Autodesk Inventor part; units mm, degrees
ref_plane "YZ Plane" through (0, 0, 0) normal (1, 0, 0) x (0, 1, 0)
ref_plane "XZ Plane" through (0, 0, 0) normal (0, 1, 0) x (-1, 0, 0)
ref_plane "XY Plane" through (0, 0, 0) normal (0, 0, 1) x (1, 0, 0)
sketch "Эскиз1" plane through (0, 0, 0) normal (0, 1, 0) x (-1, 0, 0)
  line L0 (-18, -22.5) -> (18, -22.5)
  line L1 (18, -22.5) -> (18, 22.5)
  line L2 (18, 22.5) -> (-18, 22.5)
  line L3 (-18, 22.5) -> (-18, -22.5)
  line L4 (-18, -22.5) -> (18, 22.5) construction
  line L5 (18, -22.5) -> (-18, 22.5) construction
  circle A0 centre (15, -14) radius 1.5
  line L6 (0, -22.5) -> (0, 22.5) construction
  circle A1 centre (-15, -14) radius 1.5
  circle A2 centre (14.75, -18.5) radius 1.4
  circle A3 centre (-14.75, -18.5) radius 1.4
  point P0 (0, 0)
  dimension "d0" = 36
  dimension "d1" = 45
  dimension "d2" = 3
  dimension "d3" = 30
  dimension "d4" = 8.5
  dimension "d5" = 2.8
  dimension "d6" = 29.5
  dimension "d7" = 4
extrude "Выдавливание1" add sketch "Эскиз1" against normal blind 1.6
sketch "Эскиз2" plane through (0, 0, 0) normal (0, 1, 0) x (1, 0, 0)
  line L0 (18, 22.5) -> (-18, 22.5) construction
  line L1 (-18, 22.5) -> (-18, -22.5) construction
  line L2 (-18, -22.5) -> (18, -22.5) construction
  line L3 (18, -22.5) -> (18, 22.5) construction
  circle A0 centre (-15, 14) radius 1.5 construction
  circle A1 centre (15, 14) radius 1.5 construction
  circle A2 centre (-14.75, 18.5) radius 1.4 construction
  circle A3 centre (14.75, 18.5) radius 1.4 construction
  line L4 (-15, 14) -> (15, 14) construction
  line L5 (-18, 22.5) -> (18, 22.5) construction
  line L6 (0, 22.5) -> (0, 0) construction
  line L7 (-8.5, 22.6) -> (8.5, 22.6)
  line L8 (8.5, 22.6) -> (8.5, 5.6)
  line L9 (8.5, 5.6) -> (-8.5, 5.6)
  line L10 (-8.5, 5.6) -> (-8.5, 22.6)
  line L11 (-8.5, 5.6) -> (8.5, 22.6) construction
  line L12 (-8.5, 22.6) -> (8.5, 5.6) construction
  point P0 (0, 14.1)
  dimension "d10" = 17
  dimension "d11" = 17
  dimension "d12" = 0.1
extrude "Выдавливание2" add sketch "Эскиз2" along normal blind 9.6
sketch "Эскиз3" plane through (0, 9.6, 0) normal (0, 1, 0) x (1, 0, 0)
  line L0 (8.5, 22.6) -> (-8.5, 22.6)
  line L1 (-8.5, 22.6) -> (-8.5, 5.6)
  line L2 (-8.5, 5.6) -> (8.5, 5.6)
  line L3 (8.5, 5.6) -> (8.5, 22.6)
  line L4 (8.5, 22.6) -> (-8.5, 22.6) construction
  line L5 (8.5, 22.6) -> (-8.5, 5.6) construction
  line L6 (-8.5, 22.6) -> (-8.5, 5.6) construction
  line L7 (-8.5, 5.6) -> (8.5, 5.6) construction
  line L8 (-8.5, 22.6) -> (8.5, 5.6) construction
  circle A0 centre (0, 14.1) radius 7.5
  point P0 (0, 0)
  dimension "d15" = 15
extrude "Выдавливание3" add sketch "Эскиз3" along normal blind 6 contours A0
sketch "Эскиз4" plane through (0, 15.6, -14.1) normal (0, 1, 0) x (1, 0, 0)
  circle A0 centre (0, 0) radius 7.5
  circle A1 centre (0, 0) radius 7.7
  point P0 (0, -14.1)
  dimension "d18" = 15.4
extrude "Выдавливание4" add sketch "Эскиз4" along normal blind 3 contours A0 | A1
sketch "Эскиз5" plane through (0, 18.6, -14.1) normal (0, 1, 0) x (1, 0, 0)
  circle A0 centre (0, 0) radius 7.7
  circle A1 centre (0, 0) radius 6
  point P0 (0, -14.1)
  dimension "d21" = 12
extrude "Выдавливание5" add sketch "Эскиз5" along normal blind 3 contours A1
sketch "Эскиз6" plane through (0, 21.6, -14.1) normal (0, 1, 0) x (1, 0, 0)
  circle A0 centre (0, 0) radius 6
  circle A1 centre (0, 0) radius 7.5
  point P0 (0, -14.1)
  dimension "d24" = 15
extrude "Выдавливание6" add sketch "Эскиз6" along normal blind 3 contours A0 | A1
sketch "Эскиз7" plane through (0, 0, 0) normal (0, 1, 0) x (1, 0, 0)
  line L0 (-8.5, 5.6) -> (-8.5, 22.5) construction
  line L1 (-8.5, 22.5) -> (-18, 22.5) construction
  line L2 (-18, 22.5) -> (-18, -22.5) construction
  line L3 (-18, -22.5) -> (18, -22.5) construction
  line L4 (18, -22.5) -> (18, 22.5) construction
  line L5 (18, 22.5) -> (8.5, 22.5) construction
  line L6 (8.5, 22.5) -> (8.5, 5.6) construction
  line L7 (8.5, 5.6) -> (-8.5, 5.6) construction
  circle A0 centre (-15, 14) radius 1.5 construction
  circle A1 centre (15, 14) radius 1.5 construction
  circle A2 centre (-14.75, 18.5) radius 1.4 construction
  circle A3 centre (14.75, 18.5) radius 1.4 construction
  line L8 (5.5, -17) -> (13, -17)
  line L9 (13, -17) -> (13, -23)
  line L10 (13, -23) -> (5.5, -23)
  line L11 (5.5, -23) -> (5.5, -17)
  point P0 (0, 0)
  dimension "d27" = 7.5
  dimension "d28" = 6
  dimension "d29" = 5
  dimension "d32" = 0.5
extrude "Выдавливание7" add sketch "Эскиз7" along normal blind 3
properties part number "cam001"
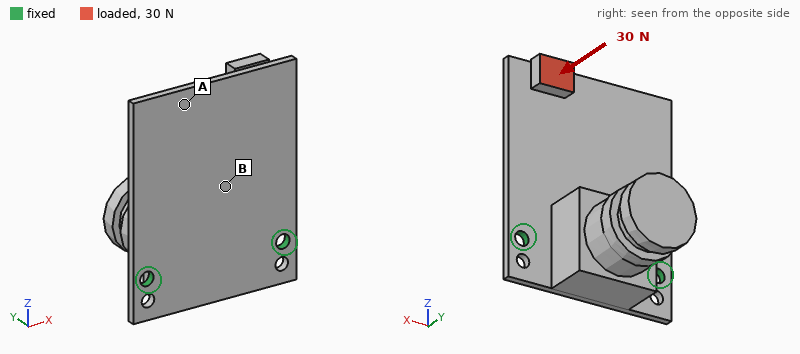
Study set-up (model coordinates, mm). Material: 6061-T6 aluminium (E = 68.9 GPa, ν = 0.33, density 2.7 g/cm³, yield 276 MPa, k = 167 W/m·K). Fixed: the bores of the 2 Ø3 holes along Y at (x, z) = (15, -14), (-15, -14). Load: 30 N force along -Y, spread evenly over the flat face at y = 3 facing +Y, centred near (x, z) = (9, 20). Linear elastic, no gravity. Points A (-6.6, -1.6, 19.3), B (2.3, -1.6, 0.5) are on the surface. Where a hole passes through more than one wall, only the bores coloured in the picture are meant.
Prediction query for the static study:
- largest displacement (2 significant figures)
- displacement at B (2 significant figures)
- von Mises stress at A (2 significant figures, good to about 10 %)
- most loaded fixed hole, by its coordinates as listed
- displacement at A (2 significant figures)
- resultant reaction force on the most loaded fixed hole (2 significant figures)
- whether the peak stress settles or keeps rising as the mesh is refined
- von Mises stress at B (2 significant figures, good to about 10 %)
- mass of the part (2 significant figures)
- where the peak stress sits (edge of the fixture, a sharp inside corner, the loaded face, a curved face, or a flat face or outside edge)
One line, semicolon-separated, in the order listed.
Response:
0.47 mm; 0.085 mm; 15 MPa; (15, -14); 0.32 mm; 29 N; keeps rising; 39 MPa; 21 g; edge of the fixture
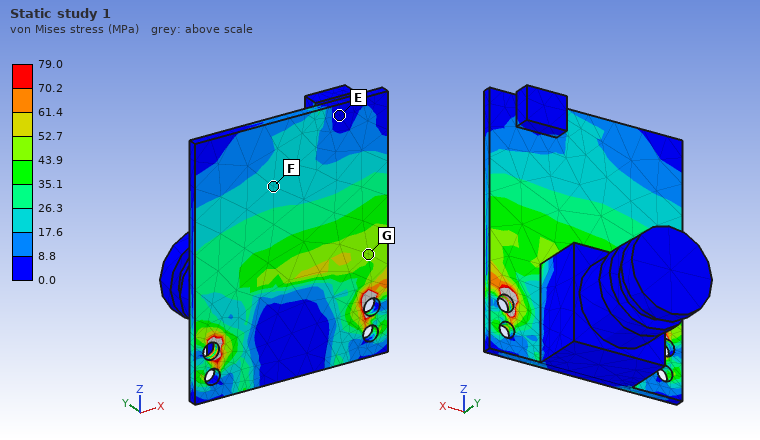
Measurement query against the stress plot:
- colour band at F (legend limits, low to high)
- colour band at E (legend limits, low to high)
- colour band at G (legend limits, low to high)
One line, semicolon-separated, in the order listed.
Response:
17.6 to 26.3 MPa; 0.0 to 8.8 MPa; 43.9 to 52.7 MPa
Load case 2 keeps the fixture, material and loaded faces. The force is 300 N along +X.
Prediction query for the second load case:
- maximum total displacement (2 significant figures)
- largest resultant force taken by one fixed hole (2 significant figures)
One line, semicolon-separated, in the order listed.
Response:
0.35 mm; 370 N
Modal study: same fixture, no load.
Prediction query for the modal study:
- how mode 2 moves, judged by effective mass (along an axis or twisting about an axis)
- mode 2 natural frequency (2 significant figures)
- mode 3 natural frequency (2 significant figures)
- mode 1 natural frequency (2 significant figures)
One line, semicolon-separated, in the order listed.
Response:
along Z; 2200 Hz; 2700 Hz; 910 Hz
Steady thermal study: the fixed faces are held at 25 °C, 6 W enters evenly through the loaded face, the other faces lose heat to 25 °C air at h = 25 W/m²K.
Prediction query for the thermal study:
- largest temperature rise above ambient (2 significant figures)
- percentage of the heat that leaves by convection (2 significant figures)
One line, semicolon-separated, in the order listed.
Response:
29 K; 17 %
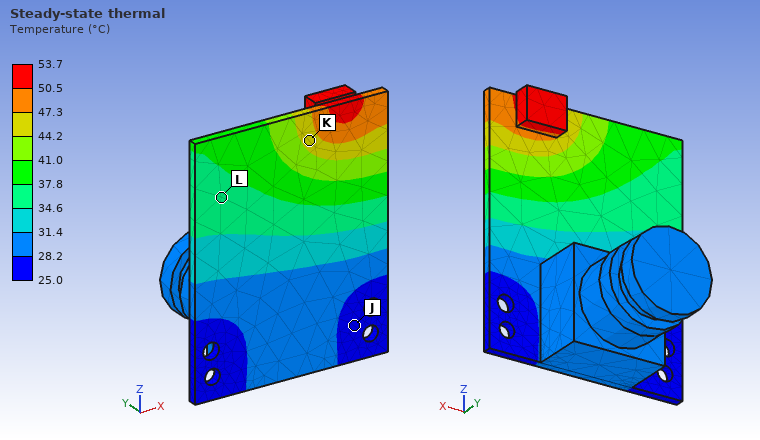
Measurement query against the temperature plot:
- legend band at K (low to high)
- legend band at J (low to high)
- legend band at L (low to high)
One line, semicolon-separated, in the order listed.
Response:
44.2 to 47.3 °C; 25.0 to 28.2 °C; 34.6 to 37.8 °C
